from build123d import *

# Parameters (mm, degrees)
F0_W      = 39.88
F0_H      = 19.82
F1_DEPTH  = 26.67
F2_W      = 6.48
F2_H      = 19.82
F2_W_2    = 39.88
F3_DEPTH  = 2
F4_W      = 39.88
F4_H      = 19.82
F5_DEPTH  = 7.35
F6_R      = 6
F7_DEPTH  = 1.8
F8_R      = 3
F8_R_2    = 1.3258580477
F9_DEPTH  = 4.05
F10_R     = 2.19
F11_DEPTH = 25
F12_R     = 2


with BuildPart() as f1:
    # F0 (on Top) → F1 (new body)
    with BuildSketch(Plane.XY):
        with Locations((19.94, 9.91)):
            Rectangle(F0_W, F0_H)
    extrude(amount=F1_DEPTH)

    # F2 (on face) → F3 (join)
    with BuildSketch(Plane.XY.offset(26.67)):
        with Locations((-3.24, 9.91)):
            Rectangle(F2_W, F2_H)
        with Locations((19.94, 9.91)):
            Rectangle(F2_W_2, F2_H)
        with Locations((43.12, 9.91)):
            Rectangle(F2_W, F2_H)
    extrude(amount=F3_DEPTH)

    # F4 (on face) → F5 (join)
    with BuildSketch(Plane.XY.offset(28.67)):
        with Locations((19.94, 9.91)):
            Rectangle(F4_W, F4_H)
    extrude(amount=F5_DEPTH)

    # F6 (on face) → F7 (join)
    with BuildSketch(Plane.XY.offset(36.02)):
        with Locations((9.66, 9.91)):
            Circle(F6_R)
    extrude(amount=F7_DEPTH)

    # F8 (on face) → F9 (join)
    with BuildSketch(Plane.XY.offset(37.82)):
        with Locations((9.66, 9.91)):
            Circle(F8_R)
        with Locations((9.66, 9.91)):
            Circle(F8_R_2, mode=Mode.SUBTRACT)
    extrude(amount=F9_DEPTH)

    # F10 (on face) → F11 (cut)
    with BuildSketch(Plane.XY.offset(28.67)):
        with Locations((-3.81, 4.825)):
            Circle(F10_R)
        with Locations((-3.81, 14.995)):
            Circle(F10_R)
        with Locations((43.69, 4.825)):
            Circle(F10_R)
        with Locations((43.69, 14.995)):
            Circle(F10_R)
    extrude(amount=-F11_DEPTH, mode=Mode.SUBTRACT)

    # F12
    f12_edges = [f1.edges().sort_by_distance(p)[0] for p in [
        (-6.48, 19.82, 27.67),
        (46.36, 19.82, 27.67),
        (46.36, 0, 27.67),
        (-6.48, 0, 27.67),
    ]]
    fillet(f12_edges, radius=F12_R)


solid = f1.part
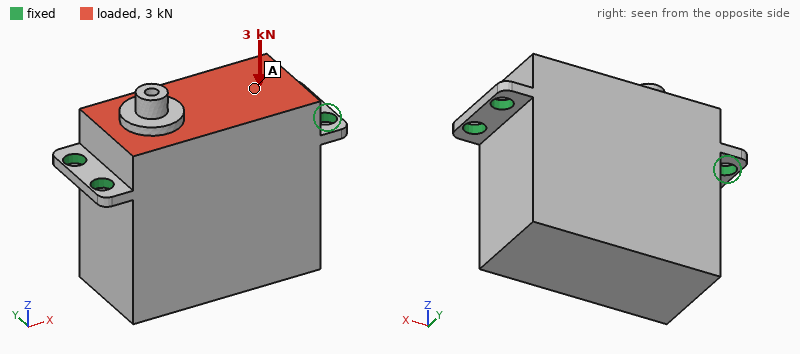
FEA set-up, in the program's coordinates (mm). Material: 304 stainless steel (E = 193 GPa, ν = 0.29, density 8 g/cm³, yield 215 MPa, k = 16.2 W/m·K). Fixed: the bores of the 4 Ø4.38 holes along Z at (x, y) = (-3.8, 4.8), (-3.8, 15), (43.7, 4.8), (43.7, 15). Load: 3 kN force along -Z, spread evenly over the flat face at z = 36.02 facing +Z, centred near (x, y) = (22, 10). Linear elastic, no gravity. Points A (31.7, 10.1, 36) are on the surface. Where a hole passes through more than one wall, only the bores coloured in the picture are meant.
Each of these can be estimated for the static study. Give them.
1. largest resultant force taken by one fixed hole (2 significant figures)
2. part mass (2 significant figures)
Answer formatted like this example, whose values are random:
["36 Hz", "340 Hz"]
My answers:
["810 N", "230 g"]
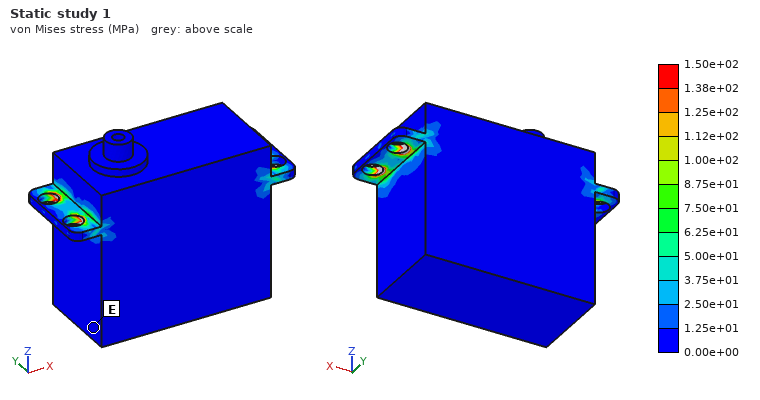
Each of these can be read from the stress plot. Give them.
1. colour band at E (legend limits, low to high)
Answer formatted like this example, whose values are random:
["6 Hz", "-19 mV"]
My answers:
["0.00e+00 to 1.25e+01 MPa"]
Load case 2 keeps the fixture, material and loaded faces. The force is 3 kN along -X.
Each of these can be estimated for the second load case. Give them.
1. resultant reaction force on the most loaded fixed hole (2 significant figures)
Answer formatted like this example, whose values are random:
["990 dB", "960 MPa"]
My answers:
["830 N"]
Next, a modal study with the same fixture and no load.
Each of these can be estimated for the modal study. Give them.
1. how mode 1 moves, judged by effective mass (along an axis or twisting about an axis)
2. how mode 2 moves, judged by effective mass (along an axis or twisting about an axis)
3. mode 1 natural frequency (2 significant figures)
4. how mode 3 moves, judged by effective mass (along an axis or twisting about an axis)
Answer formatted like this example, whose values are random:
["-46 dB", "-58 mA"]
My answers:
["along Y", "along Z", "3500 Hz", "along X"]
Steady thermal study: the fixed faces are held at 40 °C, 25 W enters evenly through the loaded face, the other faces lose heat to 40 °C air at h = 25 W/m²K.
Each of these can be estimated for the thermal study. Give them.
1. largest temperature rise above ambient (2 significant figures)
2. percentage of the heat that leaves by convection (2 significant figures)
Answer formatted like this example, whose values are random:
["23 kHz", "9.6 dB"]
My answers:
["81 K", "30 %"]
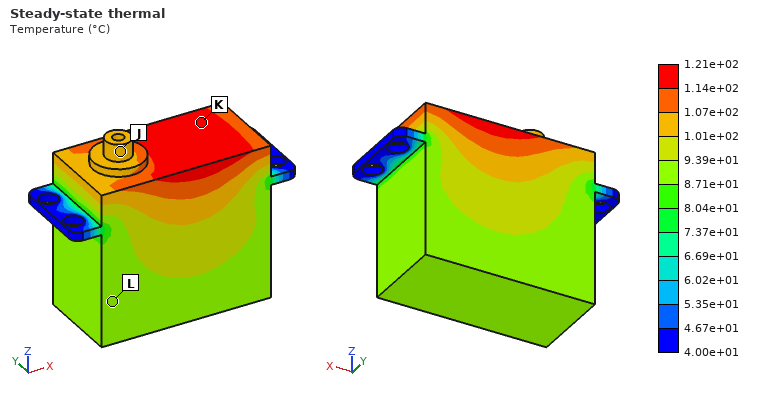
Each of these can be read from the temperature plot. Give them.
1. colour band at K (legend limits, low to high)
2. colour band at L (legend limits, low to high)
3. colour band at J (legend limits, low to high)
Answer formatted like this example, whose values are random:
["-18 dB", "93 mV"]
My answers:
["1.14e+02 to 1.21e+02 °C", "8.71e+01 to 9.39e+01 °C", "1.01e+02 to 1.07e+02 °C"]
